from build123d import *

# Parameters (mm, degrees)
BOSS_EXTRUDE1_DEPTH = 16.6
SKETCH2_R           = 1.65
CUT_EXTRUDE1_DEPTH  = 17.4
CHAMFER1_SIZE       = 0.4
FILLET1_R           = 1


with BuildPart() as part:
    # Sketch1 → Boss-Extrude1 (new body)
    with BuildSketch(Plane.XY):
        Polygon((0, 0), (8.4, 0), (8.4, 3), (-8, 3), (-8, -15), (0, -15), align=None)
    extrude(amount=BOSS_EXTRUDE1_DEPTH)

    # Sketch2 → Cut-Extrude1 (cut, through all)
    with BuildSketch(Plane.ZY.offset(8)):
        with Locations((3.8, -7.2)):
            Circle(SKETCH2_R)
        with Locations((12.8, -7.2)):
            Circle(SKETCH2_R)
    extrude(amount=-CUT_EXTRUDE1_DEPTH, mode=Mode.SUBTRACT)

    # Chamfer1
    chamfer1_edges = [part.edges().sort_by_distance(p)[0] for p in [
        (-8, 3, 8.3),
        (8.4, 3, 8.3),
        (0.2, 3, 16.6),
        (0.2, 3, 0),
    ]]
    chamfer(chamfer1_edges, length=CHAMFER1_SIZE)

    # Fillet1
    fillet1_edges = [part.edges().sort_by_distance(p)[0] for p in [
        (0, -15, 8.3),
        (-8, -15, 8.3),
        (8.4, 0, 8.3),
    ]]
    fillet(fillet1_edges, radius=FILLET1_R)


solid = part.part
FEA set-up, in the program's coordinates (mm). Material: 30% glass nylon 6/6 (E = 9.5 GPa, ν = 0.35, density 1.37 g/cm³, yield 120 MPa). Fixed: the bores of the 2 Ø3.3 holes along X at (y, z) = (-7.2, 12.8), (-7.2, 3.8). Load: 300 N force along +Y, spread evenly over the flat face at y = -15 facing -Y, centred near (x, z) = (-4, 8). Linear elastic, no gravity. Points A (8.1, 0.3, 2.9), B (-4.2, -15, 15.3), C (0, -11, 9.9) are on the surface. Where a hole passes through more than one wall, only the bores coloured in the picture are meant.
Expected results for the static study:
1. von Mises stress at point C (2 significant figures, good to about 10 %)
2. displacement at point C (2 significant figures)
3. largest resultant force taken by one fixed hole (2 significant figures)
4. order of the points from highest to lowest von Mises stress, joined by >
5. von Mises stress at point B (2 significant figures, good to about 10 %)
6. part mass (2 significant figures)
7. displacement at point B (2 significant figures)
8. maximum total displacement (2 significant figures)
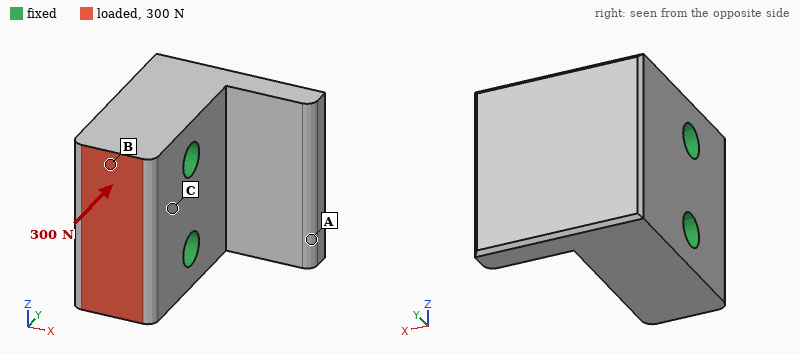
1.3 MPa
0.86 µm
150 N
B > C > A
2.6 MPa
3.6 g
2.3 µm
2.6 µm
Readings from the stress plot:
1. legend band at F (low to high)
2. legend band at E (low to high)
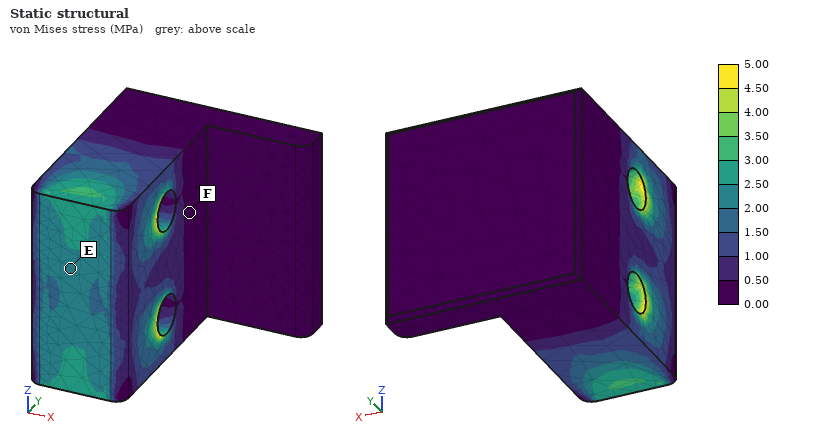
0.00 to 0.50 MPa
2.00 to 2.50 MPa
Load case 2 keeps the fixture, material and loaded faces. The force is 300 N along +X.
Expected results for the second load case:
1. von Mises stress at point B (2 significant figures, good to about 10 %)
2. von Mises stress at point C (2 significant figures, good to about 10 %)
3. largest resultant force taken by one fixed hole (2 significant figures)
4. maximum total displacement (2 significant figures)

5.3 MPa
5.4 MPa
150 N
12 µm
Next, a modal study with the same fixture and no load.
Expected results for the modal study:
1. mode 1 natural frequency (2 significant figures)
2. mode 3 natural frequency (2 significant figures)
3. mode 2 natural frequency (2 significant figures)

11 kHz
19 kHz
16 kHz
